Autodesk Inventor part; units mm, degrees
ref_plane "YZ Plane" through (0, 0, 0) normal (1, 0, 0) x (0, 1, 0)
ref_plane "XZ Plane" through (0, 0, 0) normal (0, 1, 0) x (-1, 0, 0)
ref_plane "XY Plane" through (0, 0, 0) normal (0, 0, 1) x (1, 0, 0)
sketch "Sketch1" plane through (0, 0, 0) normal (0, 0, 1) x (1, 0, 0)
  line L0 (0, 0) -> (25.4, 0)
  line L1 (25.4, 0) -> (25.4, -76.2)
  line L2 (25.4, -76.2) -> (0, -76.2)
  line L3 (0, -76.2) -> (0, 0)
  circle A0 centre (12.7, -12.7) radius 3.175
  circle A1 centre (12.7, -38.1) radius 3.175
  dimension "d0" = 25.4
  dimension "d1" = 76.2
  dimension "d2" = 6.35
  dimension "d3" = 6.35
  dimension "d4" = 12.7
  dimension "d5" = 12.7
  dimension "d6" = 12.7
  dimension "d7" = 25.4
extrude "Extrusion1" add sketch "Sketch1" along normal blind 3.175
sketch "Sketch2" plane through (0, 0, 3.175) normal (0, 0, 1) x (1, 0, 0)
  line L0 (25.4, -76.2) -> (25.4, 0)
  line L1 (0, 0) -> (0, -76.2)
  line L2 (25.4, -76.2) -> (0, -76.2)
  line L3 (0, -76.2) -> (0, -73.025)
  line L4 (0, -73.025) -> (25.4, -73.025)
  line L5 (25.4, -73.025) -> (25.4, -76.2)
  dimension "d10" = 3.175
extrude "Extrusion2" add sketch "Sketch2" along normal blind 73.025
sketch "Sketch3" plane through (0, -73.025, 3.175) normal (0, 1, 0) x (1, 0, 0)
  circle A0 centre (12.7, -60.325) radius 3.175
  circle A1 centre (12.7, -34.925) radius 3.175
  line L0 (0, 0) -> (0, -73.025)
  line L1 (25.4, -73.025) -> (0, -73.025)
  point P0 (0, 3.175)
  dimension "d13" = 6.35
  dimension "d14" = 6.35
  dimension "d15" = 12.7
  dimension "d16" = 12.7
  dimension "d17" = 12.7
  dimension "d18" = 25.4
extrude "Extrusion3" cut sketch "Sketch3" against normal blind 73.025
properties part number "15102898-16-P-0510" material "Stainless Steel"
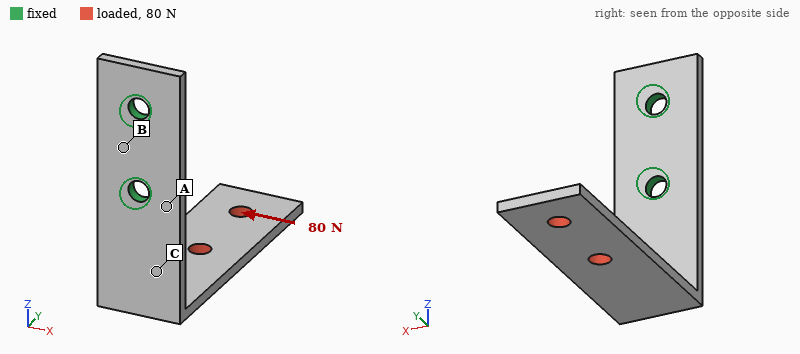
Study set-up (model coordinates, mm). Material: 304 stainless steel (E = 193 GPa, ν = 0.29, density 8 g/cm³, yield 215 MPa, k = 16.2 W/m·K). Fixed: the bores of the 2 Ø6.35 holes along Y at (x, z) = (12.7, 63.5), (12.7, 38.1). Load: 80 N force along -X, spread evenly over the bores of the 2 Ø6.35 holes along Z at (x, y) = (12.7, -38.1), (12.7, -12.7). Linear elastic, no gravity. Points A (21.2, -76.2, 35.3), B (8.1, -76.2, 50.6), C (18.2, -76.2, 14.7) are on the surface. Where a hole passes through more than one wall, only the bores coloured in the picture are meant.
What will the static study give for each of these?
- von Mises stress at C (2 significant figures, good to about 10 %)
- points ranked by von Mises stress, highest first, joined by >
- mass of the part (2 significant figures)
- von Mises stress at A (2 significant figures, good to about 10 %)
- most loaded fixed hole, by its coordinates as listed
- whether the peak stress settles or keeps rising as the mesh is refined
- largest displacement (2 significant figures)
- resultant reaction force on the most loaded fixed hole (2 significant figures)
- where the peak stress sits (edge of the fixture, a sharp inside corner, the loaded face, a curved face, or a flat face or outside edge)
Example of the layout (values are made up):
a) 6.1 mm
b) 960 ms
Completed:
a) 77 MPa
b) C > A > B
c) 93 g
d) 58 MPa
e) (12.7, 38.1)
f) keeps rising
g) 0.49 mm
h) 150 N
i) edge of the fixture
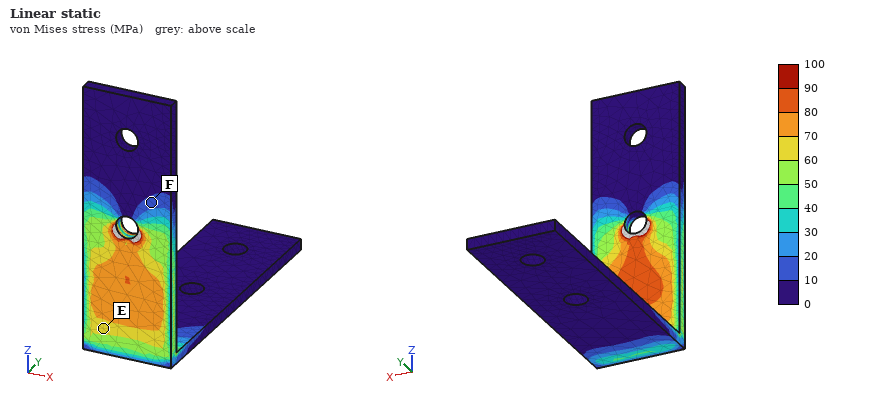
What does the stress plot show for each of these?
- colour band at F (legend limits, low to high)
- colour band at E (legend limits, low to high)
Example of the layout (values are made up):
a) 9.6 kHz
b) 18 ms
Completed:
a) 10 to 20 MPa
b) 60 to 70 MPa
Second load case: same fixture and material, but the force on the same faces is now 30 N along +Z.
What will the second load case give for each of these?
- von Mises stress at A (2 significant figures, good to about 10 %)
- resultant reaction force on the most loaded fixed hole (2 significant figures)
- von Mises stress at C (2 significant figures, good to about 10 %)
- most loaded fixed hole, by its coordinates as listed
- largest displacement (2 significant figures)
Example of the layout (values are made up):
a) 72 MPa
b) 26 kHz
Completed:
a) 21 MPa
b) 26 N
c) 32 MPa
d) (12.7, 38.1)
e) 0.45 mm
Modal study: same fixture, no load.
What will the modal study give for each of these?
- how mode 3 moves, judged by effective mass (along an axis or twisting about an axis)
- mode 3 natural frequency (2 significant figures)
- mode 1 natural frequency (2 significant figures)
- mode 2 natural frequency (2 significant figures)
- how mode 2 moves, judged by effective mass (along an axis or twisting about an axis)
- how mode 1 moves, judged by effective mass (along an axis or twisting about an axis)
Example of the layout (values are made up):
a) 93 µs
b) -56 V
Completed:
a) along Y
b) 950 Hz
c) 270 Hz
d) 420 Hz
e) along X
f) along Z
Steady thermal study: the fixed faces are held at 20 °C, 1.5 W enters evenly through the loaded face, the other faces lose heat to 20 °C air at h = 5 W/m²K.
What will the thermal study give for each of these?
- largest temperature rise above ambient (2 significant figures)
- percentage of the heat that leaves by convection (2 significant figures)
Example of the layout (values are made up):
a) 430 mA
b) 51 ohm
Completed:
a) 51 K
b) 59 %
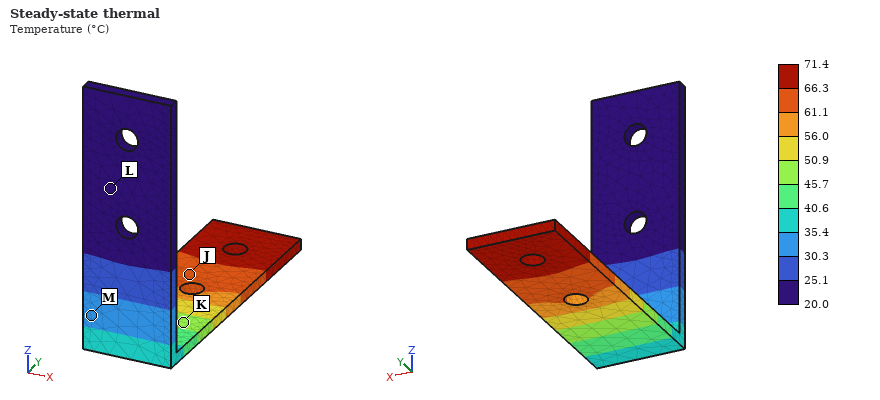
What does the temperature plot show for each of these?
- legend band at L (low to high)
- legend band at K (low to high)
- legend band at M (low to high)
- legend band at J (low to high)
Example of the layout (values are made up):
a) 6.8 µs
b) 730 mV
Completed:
a) 20.0 to 25.1 °C
b) 45.7 to 50.9 °C
c) 30.3 to 35.4 °C
d) 61.1 to 66.3 °C
